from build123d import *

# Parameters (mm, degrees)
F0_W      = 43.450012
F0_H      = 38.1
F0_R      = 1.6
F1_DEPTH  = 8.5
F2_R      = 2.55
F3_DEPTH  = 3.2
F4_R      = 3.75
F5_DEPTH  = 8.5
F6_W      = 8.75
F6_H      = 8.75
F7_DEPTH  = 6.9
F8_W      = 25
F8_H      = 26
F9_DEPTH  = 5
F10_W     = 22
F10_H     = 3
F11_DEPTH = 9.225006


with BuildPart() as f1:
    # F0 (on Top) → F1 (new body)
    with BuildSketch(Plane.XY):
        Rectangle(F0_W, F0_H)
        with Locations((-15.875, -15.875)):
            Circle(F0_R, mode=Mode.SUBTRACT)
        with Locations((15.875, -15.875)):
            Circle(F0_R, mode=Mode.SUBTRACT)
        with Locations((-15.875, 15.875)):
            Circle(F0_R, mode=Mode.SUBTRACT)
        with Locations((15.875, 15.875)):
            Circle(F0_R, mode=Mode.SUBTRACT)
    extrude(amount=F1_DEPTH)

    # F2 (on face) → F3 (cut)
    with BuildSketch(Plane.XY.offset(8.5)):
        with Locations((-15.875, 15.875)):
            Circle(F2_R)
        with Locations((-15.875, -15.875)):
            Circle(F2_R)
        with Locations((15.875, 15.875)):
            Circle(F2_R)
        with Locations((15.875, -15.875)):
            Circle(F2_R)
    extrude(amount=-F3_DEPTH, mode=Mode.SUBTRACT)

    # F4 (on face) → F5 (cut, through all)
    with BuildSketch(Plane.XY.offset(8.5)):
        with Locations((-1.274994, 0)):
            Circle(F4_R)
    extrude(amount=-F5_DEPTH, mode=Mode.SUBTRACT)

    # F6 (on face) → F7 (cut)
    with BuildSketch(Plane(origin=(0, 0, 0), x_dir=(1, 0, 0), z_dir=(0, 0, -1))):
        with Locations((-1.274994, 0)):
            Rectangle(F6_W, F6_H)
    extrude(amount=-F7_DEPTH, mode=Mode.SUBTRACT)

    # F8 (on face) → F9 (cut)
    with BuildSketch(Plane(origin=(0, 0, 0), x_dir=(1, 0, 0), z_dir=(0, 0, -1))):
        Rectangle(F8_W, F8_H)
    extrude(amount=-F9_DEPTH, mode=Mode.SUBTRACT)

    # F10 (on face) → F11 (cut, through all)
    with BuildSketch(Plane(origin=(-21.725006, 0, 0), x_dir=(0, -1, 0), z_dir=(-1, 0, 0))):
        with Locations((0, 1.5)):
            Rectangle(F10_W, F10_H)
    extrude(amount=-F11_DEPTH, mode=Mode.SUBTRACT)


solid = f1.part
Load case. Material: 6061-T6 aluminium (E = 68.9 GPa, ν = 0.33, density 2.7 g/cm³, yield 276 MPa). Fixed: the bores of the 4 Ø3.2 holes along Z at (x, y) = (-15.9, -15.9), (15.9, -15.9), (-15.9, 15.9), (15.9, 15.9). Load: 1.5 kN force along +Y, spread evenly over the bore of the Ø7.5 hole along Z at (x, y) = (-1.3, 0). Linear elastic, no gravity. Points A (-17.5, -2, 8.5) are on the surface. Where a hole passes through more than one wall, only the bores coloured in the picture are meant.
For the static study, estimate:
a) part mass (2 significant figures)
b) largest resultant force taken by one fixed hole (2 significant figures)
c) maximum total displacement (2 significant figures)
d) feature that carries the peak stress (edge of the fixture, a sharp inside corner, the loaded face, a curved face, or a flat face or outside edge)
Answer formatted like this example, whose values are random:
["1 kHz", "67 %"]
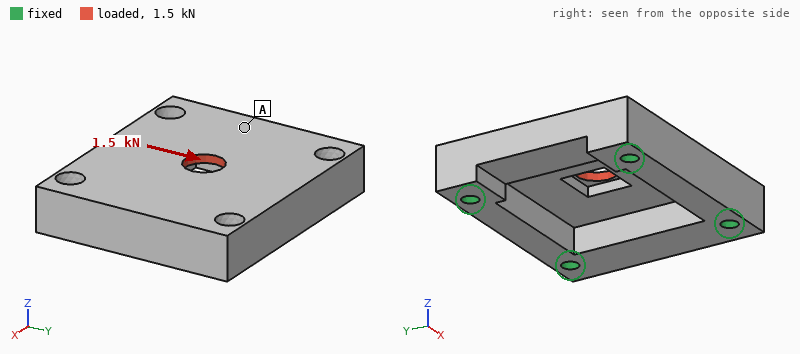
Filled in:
["26 g", "420 N", "6.7 µm", "the loaded face"]
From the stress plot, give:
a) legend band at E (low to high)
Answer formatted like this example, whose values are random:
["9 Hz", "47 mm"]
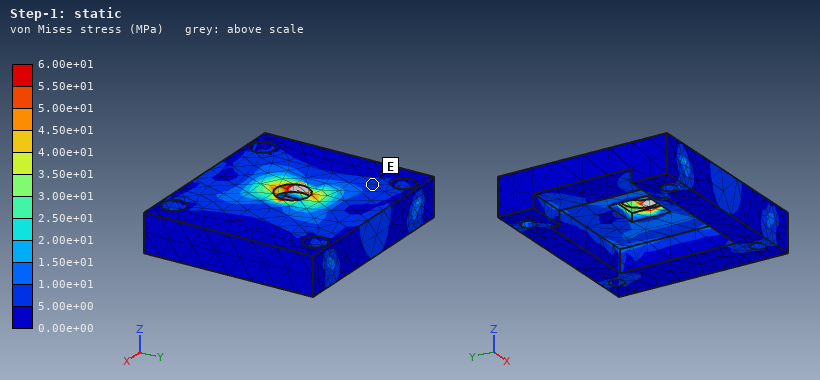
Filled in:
["5.00e+00 to 1.00e+01 MPa"]
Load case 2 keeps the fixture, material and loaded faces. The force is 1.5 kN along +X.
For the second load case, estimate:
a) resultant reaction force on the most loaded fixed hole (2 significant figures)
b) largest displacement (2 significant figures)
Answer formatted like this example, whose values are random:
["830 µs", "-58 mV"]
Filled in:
["410 N", "6.7 µm"]
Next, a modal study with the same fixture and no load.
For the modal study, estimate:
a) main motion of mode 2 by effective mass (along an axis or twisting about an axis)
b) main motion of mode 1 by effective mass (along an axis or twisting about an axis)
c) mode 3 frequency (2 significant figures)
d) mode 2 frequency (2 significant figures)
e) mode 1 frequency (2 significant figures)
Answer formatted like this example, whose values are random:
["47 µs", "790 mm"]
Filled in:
["twisting about Y", "along Z", "27 kHz", "26 kHz", "20 kHz"]
